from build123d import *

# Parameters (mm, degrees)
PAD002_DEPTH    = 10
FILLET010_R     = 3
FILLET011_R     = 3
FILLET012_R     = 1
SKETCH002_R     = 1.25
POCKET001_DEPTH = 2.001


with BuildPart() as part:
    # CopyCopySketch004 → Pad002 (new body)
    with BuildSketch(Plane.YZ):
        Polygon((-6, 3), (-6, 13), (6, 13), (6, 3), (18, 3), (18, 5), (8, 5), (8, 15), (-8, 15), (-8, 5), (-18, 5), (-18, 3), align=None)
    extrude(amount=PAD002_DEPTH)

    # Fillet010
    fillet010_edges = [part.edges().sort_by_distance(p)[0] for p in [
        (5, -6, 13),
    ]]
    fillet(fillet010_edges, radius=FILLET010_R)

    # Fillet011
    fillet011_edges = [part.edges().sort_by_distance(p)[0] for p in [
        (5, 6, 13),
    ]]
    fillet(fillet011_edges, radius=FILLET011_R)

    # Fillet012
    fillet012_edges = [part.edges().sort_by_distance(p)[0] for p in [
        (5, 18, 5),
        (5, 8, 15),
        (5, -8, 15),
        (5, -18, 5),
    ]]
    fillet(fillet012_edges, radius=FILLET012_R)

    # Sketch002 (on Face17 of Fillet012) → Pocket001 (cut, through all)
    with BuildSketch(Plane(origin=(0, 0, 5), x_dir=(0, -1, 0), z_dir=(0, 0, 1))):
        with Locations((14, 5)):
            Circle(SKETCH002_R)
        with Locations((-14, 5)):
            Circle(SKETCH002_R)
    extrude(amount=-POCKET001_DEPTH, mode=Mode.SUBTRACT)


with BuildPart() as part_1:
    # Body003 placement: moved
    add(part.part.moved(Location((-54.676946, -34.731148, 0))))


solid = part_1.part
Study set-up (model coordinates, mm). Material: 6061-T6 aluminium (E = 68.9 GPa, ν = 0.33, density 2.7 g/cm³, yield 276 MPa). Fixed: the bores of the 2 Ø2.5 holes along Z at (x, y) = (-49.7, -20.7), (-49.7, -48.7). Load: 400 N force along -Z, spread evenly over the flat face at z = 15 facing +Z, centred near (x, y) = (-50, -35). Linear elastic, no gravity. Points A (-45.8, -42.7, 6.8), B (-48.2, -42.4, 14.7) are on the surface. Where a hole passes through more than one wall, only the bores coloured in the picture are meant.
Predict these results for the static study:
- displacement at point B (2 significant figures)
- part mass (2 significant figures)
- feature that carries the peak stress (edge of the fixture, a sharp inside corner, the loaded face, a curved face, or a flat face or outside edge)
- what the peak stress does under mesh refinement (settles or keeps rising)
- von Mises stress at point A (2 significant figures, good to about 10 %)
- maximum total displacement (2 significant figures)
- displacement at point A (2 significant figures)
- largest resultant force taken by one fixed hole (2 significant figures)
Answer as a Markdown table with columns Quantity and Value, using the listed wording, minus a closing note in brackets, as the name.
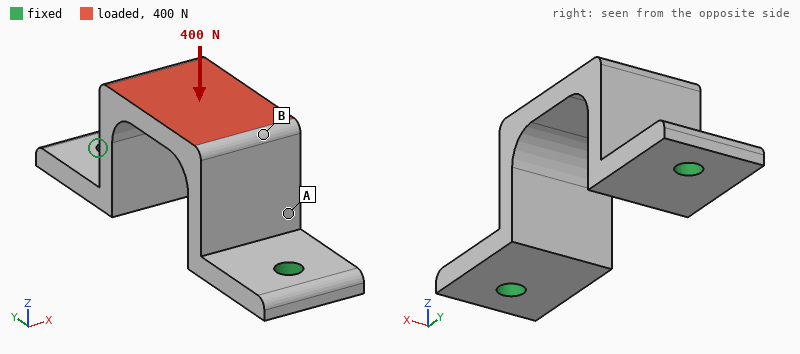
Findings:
| Quantity | Value |
|---|---|
| displacement at point B | 19 µm |
| part mass | 3.1 g |
| feature that carries the peak stress | edge of the fixture |
| what the peak stress does under mesh refinement | keeps rising |
| von Mises stress at point A | 45 MPa |
| maximum total displacement | 23 µm |
| displacement at point A | 19 µm |
| largest resultant force taken by one fixed hole | 230 N |
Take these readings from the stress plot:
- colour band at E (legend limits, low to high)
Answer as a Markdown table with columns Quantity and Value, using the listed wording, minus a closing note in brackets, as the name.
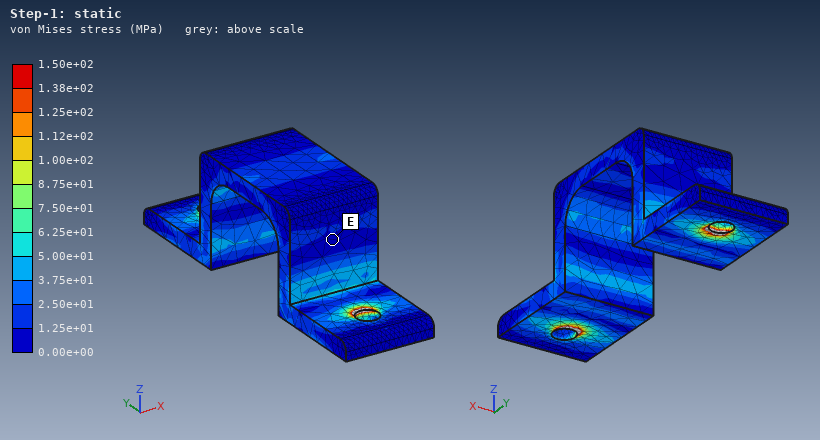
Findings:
| Quantity | Value |
|---|---|
| colour band at E | 0.00e+00 to 1.25e+01 MPa |
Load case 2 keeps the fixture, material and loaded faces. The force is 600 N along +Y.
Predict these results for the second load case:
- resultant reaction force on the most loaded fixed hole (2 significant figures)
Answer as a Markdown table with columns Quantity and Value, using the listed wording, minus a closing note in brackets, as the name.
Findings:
| Quantity | Value |
|---|---|
| resultant reaction force on the most loaded fixed hole | 410 N |
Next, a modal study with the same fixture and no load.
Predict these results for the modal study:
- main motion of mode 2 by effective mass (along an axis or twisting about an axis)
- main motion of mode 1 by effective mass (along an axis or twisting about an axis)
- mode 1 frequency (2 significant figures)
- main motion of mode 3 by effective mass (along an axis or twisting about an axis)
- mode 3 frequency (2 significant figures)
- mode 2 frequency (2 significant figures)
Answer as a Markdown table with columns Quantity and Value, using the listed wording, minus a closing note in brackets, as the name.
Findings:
| Quantity | Value |
|---|---|
| main motion of mode 2 by effective mass | along Y |
| main motion of mode 1 by effective mass | along X |
| mode 1 frequency | 6400 Hz |
| main motion of mode 3 by effective mass | along Z |
| mode 3 frequency | 15 kHz |
| mode 2 frequency | 13 kHz |
